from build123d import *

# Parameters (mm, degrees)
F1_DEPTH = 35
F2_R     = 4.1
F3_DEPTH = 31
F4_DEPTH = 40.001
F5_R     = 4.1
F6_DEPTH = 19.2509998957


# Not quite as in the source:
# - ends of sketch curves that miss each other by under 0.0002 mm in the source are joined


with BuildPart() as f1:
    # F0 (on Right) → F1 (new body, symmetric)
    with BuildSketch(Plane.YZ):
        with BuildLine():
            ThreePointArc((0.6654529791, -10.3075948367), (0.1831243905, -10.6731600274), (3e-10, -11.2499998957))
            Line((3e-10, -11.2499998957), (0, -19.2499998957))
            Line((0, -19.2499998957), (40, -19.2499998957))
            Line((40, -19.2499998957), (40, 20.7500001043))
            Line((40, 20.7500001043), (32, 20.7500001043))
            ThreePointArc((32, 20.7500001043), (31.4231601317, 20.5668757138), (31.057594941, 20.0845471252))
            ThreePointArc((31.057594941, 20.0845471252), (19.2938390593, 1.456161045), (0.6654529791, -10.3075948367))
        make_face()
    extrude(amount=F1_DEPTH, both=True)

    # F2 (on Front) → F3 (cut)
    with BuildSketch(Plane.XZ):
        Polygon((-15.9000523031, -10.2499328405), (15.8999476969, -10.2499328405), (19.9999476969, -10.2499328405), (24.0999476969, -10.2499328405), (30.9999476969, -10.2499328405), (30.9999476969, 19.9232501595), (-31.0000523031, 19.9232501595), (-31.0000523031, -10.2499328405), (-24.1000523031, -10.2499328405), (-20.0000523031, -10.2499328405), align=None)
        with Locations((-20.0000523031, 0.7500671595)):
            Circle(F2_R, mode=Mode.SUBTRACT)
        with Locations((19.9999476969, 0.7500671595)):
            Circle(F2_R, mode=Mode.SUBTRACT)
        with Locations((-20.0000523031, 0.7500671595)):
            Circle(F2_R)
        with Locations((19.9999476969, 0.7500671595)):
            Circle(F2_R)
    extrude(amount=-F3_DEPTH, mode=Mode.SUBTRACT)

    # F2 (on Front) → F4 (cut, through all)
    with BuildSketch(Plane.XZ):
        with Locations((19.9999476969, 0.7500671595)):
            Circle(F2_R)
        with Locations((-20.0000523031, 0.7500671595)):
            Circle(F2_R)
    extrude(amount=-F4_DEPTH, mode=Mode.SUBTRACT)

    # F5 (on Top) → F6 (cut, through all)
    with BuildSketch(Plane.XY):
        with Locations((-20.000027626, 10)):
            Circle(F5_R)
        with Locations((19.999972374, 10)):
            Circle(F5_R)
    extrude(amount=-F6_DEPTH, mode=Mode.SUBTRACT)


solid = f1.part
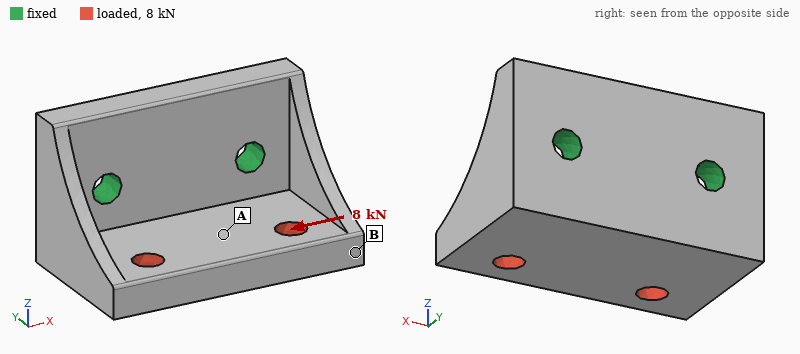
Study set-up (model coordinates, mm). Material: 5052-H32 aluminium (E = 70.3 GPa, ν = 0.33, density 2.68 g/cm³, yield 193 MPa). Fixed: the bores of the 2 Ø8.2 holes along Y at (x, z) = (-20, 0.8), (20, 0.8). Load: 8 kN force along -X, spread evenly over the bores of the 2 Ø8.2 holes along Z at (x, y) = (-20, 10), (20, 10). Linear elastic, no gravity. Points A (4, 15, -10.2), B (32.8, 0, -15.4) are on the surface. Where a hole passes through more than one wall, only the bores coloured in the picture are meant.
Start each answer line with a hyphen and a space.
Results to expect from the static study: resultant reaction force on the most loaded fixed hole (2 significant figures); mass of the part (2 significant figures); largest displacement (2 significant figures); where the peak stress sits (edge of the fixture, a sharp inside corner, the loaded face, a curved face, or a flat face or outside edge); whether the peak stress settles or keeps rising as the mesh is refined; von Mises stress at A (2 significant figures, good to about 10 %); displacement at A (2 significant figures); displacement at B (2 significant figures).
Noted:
- 6.3 kN
- 120 g
- 97 µm
- edge of the fixture
- keeps rising
- 43 MPa
- 46 µm
- 93 µm
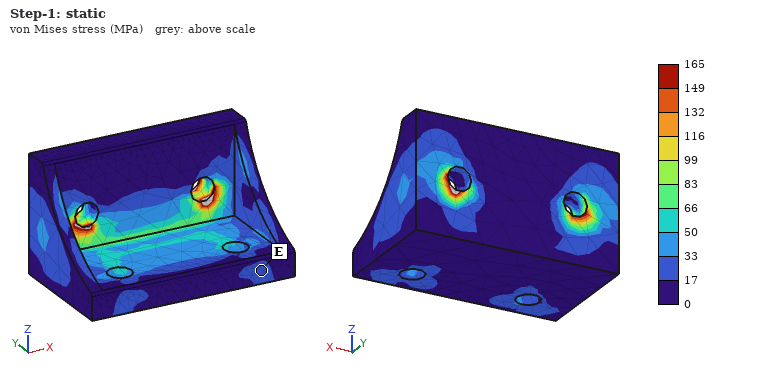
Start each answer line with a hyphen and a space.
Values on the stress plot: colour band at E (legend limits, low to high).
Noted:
- 17 to 33 MPa
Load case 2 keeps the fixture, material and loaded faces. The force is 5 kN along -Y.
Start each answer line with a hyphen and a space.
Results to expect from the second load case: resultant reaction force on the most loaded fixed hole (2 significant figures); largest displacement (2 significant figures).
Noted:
- 2.5 kN
- 61 µm
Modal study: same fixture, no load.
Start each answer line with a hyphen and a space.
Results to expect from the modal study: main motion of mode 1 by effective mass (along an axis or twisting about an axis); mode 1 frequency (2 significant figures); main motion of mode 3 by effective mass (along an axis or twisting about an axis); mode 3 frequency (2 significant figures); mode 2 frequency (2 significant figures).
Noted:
- along Z
- 4800 Hz
- along X
- 12 kHz
- 6900 Hz
